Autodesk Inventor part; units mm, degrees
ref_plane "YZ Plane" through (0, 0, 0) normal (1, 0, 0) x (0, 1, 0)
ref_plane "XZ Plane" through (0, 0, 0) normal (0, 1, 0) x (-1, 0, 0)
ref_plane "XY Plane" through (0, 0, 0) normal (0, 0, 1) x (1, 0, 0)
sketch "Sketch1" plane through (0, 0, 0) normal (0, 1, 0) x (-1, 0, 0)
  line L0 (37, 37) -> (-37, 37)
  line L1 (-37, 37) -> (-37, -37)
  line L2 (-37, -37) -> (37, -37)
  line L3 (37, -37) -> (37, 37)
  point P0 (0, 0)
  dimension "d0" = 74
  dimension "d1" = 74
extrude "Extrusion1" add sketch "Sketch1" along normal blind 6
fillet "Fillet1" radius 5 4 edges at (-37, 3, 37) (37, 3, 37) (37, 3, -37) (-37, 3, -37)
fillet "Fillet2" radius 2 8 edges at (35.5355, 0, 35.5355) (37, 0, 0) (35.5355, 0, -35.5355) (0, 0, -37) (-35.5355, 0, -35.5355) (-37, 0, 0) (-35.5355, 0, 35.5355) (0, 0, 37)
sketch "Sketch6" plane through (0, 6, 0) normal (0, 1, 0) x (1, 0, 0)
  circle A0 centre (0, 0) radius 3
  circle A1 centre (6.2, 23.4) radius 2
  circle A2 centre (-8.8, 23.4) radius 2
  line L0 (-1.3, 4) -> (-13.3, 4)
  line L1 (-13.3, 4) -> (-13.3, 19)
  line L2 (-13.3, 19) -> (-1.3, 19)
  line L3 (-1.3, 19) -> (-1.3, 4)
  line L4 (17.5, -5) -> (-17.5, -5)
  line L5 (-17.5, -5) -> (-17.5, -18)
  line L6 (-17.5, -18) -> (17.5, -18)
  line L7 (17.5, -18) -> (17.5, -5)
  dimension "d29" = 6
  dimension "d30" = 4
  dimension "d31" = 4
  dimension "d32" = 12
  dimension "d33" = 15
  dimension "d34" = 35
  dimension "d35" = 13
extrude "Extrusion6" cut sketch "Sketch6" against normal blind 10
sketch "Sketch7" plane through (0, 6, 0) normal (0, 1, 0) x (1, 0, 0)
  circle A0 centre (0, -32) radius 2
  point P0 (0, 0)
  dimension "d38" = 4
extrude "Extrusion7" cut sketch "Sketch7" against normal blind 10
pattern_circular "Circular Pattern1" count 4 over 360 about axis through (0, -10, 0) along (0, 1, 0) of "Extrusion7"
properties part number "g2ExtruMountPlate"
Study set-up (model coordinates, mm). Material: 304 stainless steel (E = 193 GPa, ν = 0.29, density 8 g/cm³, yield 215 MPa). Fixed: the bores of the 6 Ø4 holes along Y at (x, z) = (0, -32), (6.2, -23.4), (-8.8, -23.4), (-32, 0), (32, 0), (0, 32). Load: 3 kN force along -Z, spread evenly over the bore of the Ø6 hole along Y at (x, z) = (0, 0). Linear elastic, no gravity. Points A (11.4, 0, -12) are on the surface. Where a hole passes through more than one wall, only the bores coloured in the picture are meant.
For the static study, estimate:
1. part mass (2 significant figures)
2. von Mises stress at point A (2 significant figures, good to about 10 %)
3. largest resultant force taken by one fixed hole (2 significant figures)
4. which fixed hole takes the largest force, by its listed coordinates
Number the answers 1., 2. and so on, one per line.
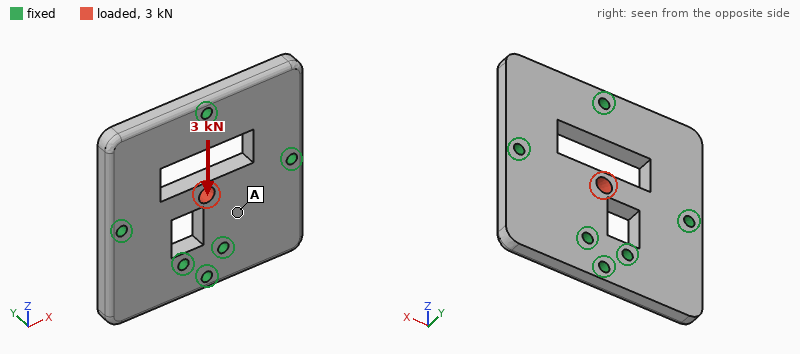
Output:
1. 220 g
2. 12 MPa
3. 1.7 kN
4. (6.2, -23.4)
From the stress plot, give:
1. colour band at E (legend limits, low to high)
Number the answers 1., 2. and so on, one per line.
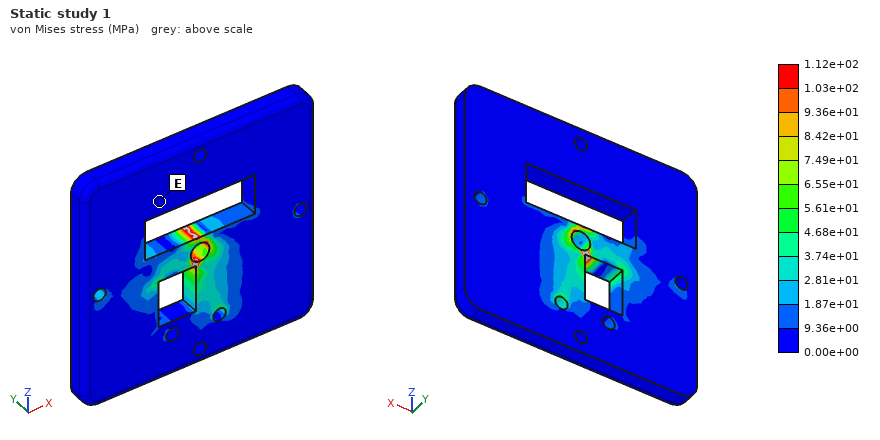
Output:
1. 0.00e+00 to 9.36e+00 MPa
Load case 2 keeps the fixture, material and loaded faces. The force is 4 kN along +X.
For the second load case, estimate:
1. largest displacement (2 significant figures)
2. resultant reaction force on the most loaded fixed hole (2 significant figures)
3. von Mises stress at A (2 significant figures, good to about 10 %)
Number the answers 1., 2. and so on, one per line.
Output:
1. 4.5 µm
2. 1.5 kN
3. 8.9 MPa
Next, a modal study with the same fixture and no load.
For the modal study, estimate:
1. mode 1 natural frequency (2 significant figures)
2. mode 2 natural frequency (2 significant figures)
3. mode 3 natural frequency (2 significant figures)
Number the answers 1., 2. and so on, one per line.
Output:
1. 6400 Hz
2. 6500 Hz
3. 7600 Hz
